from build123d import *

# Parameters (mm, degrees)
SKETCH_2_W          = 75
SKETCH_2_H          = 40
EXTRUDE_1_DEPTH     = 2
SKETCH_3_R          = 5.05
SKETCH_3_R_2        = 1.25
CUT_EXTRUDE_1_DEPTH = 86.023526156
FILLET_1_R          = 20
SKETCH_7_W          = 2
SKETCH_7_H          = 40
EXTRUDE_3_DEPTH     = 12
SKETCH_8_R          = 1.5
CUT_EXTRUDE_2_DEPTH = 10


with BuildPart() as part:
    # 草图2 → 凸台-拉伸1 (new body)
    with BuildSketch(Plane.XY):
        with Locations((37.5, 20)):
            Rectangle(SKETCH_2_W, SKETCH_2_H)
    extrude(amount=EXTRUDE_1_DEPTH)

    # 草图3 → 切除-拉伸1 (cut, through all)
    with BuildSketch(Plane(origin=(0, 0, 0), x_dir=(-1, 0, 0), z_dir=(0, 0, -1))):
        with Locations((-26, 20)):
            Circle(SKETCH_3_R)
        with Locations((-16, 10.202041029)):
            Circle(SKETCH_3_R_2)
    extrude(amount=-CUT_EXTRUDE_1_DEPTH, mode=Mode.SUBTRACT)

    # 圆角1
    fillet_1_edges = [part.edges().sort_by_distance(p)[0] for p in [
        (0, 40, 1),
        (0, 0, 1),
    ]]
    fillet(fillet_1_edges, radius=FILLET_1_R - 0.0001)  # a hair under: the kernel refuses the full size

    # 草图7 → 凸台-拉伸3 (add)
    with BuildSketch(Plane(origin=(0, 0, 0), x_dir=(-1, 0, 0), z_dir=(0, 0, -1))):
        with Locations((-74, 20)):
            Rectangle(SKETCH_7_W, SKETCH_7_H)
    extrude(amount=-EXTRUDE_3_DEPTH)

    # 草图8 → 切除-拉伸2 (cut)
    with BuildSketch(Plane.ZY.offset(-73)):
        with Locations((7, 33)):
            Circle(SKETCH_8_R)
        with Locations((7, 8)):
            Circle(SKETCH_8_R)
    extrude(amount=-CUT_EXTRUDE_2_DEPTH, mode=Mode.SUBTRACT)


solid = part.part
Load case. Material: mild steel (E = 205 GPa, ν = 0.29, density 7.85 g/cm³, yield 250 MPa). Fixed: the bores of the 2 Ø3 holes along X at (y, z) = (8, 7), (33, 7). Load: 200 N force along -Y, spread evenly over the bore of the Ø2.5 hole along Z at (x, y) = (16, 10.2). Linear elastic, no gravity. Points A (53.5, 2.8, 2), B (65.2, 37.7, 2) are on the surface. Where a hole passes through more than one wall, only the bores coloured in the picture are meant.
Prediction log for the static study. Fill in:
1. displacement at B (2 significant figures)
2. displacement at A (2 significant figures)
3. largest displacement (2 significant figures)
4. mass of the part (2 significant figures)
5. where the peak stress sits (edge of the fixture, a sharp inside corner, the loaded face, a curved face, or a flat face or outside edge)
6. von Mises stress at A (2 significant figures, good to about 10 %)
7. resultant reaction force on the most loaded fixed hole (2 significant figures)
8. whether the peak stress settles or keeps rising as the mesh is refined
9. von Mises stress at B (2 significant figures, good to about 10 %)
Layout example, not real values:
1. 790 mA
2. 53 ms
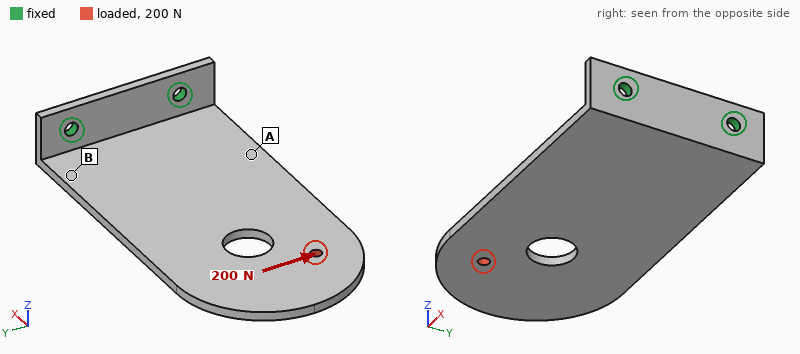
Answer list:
1. 23 µm
2. 35 µm
3. 75 µm
4. 49 g
5. edge of the fixture
6. 20 MPa
7. 450 N
8. keeps rising
9. 43 MPa
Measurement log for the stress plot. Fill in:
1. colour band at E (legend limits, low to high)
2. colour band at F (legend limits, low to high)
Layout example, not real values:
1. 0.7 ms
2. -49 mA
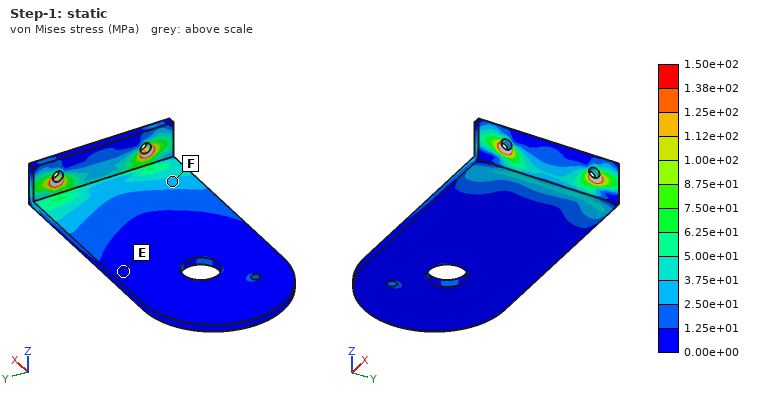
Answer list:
1. 0.00e+00 to 1.25e+01 MPa
2. 2.50e+01 to 3.75e+01 MPa
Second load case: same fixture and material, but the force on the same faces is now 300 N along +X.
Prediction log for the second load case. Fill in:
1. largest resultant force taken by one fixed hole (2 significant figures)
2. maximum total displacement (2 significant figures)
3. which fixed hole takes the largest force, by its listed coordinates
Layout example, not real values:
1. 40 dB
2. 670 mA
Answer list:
1. 270 N
2. 86 µm
3. (8, 7)
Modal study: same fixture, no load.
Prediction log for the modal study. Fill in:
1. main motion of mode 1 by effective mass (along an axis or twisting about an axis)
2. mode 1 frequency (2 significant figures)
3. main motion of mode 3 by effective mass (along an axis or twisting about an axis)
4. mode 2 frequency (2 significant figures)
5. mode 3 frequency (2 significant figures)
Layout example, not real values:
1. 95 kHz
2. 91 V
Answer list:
1. along Z
2. 300 Hz
3. along Z
4. 1300 Hz
5. 1800 Hz
